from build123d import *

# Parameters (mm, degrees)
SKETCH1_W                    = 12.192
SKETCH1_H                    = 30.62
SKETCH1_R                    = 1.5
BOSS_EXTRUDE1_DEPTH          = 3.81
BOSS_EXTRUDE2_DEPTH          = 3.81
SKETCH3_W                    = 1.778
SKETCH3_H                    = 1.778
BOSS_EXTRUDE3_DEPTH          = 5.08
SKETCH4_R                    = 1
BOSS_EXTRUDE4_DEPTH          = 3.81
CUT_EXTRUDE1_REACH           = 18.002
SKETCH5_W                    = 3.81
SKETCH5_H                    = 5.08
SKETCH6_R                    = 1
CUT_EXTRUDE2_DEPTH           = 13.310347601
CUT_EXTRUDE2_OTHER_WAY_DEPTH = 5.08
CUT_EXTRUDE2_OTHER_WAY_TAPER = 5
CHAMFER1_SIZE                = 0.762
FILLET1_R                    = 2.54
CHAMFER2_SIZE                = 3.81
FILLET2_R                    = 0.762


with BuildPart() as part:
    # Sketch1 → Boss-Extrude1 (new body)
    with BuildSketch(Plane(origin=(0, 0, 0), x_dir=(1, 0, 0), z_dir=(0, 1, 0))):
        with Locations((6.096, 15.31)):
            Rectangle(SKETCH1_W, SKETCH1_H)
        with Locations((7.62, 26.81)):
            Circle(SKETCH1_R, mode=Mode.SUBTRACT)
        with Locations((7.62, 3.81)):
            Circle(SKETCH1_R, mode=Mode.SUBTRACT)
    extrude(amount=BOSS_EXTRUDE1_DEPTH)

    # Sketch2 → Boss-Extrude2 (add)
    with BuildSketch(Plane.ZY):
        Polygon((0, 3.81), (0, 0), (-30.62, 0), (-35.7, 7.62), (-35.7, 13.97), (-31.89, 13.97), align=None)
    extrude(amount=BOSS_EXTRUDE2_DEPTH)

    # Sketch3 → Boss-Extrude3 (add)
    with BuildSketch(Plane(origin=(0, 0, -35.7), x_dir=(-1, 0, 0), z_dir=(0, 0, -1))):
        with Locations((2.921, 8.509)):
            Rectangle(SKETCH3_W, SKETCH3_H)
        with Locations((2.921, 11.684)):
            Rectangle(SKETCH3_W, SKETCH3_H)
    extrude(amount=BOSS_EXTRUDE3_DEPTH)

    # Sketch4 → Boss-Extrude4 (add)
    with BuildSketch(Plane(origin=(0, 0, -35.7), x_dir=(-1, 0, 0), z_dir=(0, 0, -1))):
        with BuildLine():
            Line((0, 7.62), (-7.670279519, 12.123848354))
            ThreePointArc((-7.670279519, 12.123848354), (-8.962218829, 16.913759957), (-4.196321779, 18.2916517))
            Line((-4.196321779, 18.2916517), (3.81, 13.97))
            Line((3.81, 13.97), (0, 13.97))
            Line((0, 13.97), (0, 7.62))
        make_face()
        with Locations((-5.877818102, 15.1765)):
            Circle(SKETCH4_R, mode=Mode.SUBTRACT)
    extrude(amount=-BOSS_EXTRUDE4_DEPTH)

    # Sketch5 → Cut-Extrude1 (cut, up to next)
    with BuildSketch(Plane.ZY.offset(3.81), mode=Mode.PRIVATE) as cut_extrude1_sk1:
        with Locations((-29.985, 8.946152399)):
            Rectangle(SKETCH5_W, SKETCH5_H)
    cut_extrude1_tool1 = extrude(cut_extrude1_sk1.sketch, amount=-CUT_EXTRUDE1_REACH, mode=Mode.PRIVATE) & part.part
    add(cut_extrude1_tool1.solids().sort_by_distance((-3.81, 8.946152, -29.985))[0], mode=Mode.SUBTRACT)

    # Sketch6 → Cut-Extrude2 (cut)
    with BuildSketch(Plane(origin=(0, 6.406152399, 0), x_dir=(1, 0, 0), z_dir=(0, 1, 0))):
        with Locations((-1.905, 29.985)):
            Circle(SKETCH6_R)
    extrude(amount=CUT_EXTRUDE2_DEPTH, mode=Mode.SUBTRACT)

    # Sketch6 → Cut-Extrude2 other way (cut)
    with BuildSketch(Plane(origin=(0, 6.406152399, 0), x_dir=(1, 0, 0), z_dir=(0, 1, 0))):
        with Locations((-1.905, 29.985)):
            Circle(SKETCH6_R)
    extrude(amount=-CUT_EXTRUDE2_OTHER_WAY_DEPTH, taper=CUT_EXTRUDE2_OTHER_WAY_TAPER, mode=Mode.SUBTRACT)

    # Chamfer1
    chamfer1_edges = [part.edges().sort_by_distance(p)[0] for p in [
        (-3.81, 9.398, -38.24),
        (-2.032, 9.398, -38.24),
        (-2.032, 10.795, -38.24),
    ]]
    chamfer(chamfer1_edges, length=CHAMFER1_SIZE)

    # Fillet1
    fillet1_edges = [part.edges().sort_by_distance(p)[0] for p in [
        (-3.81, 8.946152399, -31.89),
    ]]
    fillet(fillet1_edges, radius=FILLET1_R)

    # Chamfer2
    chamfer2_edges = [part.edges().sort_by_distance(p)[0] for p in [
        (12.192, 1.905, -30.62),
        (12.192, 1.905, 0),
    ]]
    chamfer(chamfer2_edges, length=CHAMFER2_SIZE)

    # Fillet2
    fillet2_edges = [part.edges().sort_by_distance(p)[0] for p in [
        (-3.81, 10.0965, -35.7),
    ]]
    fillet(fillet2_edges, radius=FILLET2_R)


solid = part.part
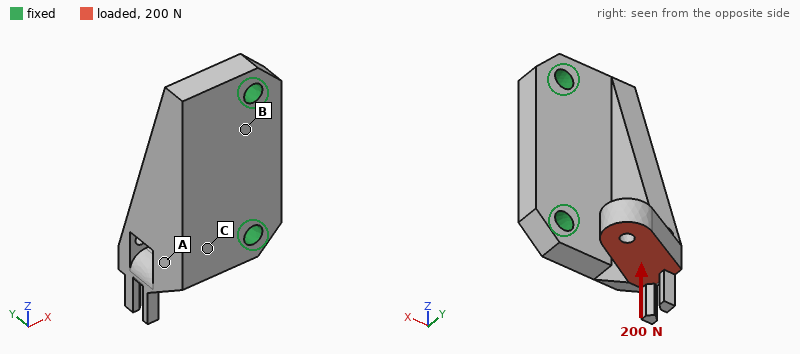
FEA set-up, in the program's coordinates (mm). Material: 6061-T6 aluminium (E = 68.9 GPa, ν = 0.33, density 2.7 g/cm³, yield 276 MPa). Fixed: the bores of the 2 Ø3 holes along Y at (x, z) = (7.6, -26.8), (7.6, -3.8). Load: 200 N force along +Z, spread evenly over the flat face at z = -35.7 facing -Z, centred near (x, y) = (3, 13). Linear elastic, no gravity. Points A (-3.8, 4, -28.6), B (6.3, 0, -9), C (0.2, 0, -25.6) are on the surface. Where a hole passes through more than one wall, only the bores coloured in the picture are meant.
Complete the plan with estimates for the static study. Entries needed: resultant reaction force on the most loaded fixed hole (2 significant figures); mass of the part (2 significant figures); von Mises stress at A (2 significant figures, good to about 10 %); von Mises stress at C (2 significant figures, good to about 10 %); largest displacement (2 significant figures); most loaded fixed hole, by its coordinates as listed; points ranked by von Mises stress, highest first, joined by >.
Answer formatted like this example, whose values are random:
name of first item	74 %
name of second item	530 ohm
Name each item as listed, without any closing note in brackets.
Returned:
resultant reaction force on the most loaded fixed hole	170 N
mass of the part	7.3 g
von Mises stress at A	43 MPa
von Mises stress at C	22 MPa
largest displacement	0.11 mm
most loaded fixed hole, by its coordinates as listed	(7.6, -26.8)
points ranked by von Mises stress, highest first, joined by >	A > C > B
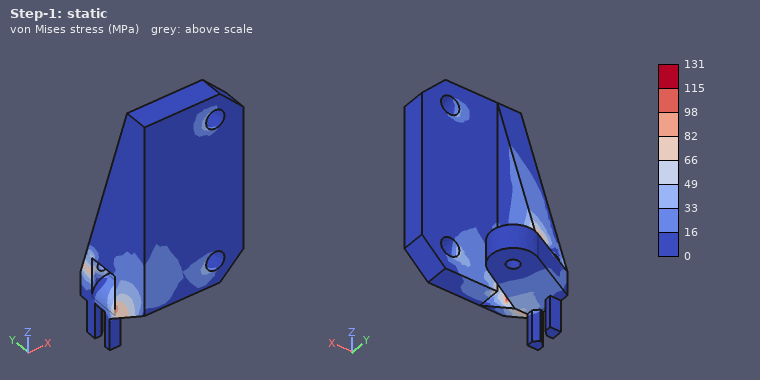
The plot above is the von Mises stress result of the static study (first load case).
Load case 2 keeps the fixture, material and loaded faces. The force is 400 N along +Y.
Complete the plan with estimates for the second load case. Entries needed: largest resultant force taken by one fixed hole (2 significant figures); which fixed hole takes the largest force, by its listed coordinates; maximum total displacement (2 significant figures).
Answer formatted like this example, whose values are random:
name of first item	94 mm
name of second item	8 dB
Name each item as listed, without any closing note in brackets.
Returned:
largest resultant force taken by one fixed hole	540 N
which fixed hole takes the largest force, by its listed coordinates	(7.6, -26.8)
maximum total displacement	0.16 mm
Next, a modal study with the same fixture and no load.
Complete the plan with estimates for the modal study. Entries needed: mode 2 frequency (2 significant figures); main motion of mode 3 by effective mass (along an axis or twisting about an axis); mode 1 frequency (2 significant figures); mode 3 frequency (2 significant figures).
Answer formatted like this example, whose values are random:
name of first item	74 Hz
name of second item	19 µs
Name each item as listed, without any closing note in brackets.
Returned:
mode 2 frequency	9300 Hz
main motion of mode 3 by effective mass	along Y
mode 1 frequency	5600 Hz
mode 3 frequency	11 kHz
